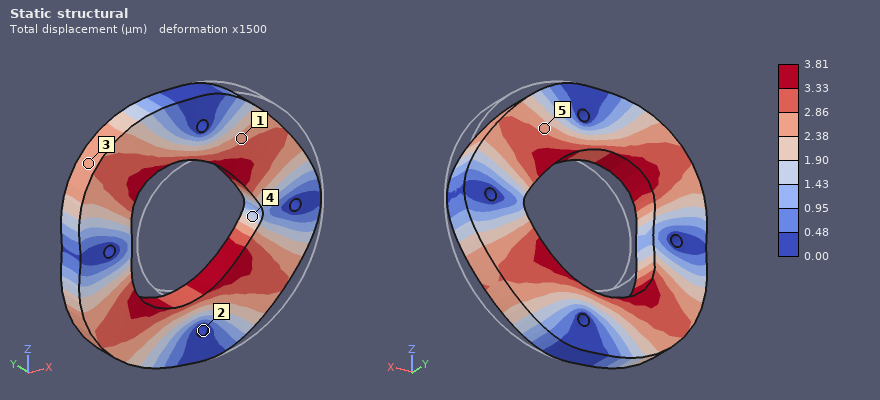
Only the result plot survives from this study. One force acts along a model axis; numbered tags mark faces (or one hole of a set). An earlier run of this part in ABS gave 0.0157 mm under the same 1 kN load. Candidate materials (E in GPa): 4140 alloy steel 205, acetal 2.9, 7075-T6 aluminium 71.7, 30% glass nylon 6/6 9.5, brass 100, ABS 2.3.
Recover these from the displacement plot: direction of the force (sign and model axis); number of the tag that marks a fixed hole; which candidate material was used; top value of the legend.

-X
2
30% glass nylon 6/6
3.81 µm
